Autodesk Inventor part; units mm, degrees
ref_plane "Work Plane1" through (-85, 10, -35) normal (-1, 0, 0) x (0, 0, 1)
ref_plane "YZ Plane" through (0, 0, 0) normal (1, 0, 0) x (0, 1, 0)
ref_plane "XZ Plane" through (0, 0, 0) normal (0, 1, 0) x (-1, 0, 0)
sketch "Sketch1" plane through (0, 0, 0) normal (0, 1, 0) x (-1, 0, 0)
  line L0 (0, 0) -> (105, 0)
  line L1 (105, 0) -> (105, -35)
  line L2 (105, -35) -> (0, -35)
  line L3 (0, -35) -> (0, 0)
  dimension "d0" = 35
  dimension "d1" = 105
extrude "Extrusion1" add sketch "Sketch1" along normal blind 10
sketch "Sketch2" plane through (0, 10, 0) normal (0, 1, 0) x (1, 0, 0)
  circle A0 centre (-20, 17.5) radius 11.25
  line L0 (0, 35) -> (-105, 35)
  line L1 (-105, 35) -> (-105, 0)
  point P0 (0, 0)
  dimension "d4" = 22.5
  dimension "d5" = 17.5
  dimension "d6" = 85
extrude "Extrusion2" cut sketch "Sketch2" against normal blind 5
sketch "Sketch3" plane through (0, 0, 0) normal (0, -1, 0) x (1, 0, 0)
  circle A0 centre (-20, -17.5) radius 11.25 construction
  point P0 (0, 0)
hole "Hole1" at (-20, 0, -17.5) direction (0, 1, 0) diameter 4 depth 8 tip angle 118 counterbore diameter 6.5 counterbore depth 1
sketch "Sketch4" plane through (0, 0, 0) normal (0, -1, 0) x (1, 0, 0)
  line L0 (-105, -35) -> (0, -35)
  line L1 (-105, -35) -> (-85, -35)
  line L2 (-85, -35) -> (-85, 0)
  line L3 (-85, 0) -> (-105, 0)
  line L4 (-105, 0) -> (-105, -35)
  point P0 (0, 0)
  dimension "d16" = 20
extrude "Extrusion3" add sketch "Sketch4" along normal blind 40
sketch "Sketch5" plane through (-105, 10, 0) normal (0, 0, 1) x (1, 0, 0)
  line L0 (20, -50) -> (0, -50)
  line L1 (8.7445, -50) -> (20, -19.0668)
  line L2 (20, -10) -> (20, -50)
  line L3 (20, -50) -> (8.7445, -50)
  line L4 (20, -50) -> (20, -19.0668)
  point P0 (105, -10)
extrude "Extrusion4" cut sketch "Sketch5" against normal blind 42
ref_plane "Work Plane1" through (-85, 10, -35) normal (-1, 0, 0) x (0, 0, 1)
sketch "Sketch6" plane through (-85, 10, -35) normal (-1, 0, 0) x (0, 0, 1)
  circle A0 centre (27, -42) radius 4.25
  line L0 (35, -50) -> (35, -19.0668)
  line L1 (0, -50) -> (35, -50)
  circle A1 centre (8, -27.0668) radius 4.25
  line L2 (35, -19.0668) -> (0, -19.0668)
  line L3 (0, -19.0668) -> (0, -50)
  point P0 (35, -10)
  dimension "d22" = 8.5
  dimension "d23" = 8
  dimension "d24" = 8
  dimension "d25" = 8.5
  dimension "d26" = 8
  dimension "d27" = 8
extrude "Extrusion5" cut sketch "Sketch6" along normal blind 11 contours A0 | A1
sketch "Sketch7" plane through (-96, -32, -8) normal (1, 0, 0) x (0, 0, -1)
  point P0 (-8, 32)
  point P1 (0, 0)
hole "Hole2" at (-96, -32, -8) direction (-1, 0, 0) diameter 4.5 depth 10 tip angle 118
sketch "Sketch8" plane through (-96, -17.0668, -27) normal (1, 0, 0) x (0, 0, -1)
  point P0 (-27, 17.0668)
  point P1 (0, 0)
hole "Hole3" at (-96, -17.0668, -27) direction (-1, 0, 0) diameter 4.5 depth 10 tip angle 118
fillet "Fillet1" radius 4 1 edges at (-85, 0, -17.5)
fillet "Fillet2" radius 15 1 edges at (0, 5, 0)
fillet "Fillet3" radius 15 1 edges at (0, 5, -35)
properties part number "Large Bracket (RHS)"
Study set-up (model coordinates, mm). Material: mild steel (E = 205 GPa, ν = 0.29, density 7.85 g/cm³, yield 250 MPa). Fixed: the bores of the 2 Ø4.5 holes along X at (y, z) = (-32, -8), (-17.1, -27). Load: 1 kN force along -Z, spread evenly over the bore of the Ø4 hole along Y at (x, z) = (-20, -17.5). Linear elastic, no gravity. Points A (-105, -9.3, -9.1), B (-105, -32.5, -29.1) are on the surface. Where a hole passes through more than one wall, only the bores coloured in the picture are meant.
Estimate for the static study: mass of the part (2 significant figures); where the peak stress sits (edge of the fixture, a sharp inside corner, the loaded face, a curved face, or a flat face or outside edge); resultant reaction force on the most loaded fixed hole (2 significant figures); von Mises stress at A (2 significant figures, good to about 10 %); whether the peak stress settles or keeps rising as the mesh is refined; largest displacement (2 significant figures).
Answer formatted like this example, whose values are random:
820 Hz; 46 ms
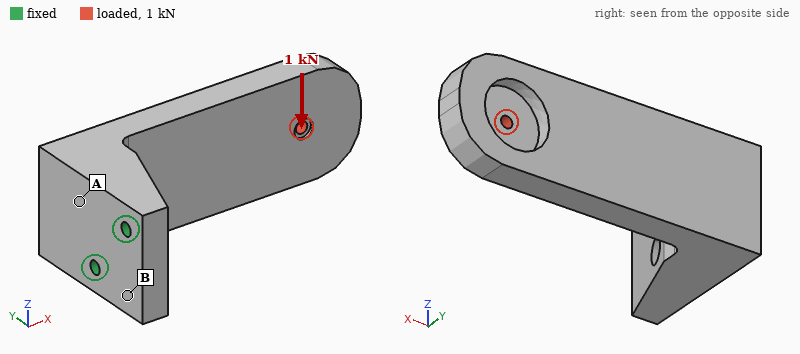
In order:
430 g; edge of the fixture; 2.6 kN; 29 MPa; keeps rising; 0.11 mm
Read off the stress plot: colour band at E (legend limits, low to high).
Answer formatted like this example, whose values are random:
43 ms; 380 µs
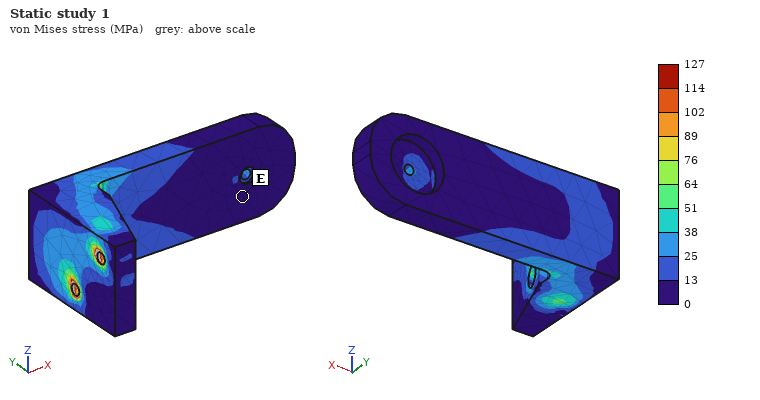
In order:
0 to 13 MPa
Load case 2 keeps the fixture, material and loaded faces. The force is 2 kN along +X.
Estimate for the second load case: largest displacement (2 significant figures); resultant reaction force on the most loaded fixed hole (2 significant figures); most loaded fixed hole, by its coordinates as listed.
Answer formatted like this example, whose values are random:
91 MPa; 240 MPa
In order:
40 µm; 2.1 kN; (-17.1, -27)
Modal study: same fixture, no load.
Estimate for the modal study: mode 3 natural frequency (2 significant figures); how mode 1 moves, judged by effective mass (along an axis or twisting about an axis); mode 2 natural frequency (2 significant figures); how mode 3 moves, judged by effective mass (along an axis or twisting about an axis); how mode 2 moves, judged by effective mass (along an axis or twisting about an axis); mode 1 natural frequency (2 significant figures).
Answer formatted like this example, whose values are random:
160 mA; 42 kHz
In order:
3800 Hz; along Y; 1700 Hz; along X; along Z; 970 Hz
